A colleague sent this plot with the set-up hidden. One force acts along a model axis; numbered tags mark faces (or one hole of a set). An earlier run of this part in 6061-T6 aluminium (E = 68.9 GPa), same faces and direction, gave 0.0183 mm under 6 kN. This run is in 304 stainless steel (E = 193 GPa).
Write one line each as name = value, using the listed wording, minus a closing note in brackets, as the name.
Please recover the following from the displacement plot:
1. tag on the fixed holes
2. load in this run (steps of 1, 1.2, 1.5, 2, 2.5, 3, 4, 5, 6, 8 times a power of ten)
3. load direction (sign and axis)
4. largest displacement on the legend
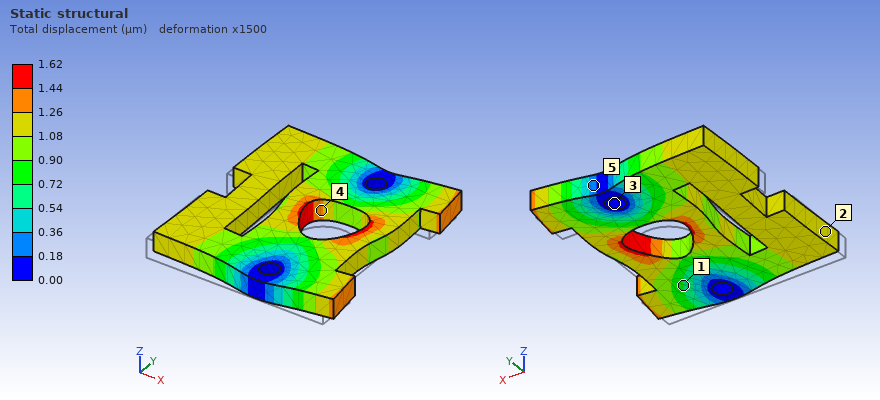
tag on the fixed holes = 3
load in this run = 1.5 kN
load direction = +Y
largest displacement on the legend = 1.62 µm
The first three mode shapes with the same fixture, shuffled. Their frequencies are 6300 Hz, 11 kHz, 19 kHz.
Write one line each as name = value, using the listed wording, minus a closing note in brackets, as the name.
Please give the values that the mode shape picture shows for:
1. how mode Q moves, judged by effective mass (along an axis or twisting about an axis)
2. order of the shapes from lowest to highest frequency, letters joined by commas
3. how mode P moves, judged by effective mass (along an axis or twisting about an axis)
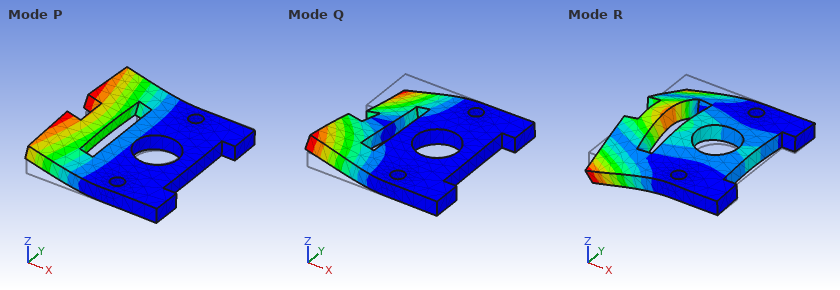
how mode Q moves, judged by effective mass = twisting about X
order of the shapes from lowest to highest frequency, letters joined by commas = P, Q, R
how mode P moves, judged by effective mass = along Z
